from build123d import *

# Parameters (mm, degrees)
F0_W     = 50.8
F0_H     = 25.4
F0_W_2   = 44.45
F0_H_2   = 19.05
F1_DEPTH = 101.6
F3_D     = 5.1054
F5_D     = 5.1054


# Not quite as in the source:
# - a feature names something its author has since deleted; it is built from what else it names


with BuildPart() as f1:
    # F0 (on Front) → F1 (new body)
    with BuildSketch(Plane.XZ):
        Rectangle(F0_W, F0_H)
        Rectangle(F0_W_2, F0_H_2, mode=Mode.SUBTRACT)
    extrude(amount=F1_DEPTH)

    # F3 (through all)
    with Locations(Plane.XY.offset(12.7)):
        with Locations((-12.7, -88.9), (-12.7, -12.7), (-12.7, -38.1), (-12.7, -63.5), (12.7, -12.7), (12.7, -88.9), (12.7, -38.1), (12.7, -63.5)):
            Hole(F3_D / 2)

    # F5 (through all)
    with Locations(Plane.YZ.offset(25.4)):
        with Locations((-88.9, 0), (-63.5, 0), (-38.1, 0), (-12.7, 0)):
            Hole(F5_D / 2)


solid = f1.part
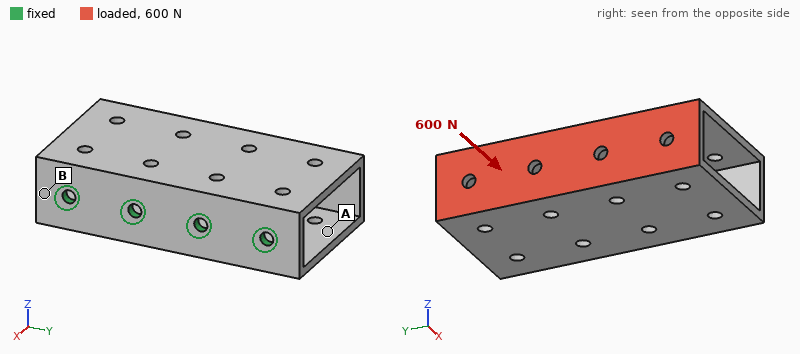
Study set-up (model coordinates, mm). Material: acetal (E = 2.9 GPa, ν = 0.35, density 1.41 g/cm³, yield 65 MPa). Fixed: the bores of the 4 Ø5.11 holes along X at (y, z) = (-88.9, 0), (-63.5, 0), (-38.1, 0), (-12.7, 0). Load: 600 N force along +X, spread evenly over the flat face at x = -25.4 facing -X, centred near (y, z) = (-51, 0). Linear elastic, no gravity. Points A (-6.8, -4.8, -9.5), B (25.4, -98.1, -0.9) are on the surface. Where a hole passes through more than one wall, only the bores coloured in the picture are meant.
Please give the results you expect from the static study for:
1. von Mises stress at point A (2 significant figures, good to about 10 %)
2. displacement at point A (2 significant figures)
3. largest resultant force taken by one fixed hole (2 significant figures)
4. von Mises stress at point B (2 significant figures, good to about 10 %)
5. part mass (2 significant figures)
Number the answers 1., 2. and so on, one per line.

1. 3.1 MPa
2. 0.18 mm
3. 150 N
4. 8.1 MPa
5. 61 g
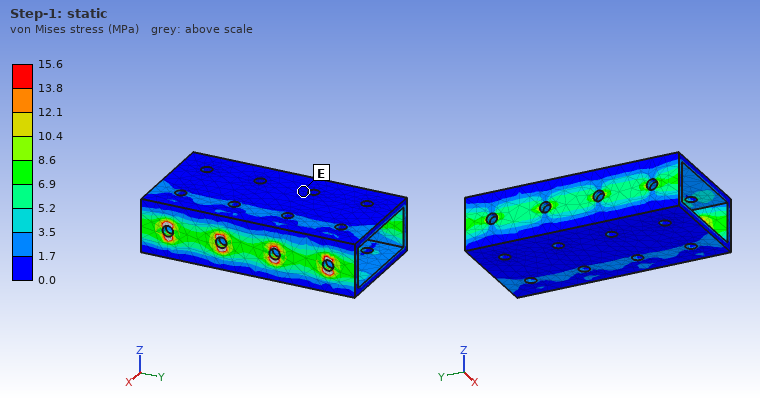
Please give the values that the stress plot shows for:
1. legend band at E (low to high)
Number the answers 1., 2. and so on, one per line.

1. 0.0 to 1.7 MPa
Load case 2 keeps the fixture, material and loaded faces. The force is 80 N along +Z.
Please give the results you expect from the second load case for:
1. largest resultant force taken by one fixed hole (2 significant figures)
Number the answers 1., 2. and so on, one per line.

1. 23 N
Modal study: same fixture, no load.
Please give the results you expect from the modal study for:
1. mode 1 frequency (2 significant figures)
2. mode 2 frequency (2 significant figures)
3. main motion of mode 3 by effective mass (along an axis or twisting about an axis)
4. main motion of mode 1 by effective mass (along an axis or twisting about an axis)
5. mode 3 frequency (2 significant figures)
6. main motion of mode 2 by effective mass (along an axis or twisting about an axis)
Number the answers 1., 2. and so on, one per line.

1. 260 Hz
2. 770 Hz
3. along Y
4. along Z
5. 1000 Hz
6. twisting about X
